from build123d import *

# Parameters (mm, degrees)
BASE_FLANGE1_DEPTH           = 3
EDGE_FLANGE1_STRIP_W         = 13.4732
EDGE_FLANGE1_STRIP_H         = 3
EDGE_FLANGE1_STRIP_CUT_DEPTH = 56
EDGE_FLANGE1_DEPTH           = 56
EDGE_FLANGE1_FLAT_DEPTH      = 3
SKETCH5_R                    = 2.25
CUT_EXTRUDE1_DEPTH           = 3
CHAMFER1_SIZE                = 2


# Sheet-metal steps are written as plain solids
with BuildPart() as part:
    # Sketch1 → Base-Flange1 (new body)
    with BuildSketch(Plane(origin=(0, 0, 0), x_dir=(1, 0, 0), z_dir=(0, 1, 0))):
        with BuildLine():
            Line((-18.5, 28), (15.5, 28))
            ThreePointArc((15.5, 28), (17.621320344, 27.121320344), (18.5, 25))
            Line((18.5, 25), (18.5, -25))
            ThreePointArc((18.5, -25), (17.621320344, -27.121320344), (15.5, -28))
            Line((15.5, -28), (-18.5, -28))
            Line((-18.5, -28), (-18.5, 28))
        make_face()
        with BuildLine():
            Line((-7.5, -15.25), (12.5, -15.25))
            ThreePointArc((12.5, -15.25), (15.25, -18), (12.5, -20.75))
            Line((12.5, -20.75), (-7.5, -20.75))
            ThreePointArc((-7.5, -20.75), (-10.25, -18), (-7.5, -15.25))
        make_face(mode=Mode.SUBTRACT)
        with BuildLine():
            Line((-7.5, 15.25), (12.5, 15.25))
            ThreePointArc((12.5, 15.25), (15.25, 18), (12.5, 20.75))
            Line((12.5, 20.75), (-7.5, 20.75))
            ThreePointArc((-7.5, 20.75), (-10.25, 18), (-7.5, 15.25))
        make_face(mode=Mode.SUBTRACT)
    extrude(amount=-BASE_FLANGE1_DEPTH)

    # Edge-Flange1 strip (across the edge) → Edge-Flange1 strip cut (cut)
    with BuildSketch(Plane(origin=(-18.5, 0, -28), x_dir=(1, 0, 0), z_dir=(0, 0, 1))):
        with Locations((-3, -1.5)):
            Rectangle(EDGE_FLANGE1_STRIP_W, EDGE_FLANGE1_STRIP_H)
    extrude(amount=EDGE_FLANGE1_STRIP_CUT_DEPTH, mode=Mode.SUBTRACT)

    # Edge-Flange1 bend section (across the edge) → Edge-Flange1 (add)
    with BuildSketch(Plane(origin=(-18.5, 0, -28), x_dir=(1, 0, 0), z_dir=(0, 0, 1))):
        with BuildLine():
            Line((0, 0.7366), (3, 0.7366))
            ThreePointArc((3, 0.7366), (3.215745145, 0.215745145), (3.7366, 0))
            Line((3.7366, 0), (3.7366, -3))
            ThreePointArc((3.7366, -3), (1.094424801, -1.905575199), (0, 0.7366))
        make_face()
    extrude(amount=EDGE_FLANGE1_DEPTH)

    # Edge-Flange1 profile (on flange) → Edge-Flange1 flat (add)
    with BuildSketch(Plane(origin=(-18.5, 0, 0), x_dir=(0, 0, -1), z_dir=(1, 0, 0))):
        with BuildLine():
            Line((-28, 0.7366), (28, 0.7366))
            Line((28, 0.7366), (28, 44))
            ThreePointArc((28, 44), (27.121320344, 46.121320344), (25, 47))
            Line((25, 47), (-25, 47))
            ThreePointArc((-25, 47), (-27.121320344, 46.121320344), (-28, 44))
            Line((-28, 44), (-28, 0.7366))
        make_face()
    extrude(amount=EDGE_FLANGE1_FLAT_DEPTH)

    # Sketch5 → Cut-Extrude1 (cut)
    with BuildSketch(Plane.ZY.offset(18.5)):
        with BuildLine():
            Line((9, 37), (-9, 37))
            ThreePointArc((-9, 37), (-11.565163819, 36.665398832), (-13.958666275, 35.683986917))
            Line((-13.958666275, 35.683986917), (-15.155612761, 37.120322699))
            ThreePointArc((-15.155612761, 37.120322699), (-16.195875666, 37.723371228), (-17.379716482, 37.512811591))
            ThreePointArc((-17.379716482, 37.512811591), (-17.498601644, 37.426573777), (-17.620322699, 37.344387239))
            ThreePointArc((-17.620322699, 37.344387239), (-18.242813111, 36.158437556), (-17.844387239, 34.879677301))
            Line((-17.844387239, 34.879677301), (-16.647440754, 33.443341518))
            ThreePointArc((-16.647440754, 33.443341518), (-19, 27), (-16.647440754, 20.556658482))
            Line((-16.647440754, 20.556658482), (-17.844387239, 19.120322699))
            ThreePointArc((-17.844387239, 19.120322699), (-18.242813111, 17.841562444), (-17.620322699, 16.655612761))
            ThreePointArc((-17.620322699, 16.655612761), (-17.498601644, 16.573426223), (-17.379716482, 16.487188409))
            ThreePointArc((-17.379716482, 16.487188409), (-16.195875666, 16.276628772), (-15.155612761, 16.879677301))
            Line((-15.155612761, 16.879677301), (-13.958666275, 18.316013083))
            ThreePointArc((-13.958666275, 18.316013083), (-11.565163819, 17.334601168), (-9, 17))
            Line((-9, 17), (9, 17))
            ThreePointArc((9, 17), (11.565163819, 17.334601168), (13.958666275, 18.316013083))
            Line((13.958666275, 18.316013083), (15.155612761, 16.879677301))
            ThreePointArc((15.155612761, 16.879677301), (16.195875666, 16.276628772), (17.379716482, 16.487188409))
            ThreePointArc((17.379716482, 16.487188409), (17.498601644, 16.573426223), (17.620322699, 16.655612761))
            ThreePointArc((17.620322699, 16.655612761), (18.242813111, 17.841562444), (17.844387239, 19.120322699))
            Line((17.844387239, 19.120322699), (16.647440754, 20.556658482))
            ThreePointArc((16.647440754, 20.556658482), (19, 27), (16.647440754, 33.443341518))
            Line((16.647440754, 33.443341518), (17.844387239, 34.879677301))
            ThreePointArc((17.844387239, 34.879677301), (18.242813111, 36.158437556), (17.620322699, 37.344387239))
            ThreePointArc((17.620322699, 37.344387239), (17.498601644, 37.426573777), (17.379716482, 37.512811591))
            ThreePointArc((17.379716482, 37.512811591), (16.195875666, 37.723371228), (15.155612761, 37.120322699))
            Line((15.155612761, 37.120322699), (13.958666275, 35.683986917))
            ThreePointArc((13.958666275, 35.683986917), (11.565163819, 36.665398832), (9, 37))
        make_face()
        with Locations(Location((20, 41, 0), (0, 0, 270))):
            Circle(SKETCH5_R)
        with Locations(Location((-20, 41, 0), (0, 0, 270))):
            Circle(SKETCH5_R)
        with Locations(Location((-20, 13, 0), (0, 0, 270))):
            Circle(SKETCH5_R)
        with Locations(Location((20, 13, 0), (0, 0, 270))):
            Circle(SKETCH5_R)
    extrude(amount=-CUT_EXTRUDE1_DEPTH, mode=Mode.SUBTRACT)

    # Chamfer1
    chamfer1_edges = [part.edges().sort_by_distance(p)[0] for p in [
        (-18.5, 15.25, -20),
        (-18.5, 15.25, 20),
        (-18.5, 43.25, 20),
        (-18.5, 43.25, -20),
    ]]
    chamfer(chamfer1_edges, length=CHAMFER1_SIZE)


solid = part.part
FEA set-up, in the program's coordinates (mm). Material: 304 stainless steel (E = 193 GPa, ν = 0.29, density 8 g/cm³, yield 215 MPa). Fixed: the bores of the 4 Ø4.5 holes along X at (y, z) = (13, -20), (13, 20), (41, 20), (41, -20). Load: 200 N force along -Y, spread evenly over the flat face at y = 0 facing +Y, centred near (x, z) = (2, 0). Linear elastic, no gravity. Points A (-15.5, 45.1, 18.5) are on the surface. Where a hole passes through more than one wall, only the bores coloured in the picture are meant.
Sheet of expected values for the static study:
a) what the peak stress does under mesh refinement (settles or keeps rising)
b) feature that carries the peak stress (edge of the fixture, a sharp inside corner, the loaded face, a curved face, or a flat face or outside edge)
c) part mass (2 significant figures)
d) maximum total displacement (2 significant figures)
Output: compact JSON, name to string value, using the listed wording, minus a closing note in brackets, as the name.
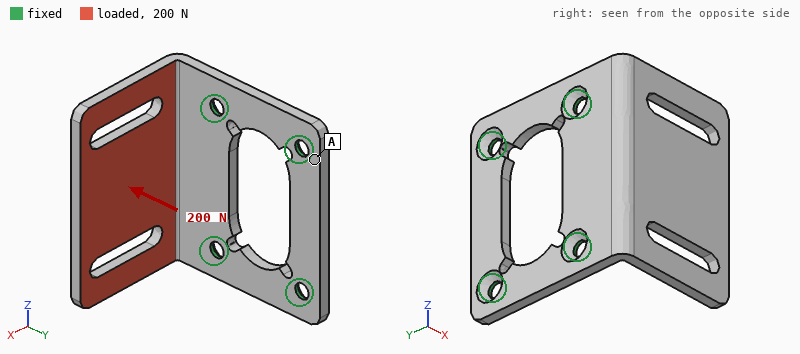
{"what the peak stress does under mesh refinement": "keeps rising", "feature that carries the peak stress": "edge of the fixture", "part mass": "85 g", "maximum total displacement": "0.18 mm"}
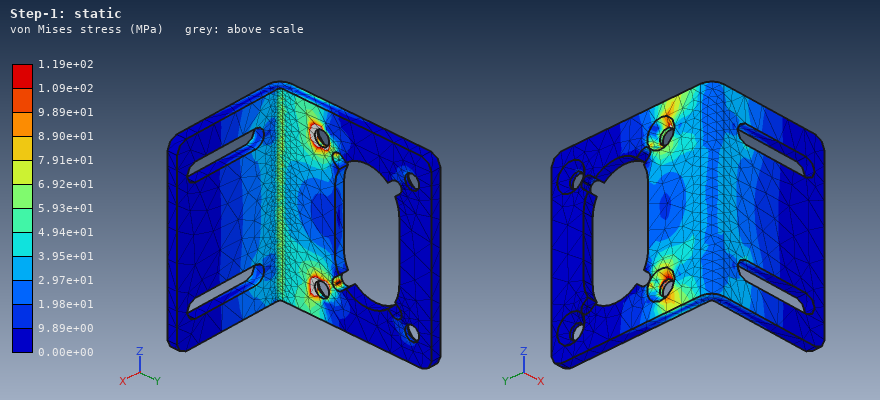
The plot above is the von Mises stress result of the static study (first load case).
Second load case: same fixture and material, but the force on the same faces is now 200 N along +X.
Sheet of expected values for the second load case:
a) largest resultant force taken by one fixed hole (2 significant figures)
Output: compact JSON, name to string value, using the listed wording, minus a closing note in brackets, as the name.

{"largest resultant force taken by one fixed hole": "130 N"}
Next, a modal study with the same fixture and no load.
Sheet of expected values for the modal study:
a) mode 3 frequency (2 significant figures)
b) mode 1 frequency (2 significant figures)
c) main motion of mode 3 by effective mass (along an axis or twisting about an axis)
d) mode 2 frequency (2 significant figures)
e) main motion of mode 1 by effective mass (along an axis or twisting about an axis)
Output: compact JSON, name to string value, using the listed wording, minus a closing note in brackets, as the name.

{"mode 3 frequency": "3500 Hz", "mode 1 frequency": "1000 Hz", "main motion of mode 3 by effective mass": "along X", "mode 2 frequency": "2400 Hz", "main motion of mode 1 by effective mass": "along Y"}
